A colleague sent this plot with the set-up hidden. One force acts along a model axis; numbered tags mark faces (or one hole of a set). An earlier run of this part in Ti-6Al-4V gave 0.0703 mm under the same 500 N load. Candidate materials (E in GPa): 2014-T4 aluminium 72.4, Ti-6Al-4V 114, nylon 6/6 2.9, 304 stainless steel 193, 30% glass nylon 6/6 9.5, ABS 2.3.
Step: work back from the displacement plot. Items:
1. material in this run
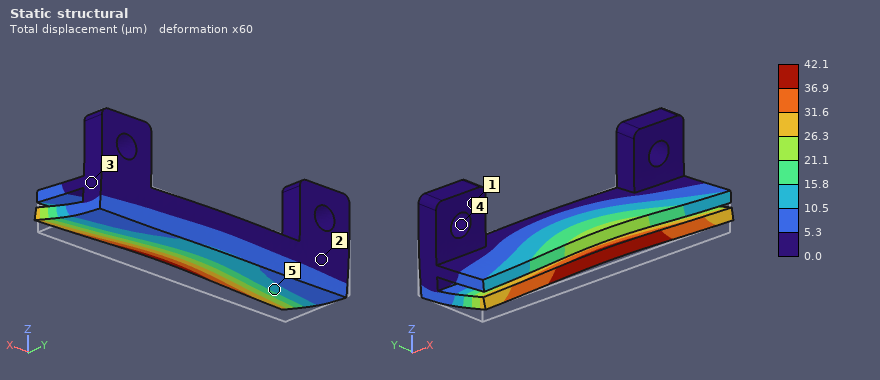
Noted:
304 stainless steel
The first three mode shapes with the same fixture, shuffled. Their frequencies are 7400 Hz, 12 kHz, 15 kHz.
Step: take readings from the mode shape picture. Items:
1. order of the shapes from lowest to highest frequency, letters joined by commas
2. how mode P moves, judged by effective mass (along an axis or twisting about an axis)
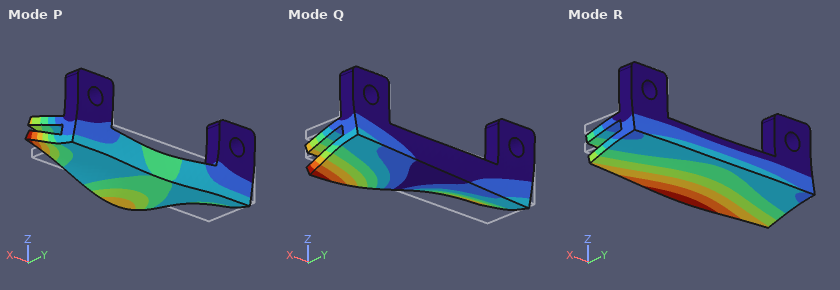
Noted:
R, Q, P
along Y
